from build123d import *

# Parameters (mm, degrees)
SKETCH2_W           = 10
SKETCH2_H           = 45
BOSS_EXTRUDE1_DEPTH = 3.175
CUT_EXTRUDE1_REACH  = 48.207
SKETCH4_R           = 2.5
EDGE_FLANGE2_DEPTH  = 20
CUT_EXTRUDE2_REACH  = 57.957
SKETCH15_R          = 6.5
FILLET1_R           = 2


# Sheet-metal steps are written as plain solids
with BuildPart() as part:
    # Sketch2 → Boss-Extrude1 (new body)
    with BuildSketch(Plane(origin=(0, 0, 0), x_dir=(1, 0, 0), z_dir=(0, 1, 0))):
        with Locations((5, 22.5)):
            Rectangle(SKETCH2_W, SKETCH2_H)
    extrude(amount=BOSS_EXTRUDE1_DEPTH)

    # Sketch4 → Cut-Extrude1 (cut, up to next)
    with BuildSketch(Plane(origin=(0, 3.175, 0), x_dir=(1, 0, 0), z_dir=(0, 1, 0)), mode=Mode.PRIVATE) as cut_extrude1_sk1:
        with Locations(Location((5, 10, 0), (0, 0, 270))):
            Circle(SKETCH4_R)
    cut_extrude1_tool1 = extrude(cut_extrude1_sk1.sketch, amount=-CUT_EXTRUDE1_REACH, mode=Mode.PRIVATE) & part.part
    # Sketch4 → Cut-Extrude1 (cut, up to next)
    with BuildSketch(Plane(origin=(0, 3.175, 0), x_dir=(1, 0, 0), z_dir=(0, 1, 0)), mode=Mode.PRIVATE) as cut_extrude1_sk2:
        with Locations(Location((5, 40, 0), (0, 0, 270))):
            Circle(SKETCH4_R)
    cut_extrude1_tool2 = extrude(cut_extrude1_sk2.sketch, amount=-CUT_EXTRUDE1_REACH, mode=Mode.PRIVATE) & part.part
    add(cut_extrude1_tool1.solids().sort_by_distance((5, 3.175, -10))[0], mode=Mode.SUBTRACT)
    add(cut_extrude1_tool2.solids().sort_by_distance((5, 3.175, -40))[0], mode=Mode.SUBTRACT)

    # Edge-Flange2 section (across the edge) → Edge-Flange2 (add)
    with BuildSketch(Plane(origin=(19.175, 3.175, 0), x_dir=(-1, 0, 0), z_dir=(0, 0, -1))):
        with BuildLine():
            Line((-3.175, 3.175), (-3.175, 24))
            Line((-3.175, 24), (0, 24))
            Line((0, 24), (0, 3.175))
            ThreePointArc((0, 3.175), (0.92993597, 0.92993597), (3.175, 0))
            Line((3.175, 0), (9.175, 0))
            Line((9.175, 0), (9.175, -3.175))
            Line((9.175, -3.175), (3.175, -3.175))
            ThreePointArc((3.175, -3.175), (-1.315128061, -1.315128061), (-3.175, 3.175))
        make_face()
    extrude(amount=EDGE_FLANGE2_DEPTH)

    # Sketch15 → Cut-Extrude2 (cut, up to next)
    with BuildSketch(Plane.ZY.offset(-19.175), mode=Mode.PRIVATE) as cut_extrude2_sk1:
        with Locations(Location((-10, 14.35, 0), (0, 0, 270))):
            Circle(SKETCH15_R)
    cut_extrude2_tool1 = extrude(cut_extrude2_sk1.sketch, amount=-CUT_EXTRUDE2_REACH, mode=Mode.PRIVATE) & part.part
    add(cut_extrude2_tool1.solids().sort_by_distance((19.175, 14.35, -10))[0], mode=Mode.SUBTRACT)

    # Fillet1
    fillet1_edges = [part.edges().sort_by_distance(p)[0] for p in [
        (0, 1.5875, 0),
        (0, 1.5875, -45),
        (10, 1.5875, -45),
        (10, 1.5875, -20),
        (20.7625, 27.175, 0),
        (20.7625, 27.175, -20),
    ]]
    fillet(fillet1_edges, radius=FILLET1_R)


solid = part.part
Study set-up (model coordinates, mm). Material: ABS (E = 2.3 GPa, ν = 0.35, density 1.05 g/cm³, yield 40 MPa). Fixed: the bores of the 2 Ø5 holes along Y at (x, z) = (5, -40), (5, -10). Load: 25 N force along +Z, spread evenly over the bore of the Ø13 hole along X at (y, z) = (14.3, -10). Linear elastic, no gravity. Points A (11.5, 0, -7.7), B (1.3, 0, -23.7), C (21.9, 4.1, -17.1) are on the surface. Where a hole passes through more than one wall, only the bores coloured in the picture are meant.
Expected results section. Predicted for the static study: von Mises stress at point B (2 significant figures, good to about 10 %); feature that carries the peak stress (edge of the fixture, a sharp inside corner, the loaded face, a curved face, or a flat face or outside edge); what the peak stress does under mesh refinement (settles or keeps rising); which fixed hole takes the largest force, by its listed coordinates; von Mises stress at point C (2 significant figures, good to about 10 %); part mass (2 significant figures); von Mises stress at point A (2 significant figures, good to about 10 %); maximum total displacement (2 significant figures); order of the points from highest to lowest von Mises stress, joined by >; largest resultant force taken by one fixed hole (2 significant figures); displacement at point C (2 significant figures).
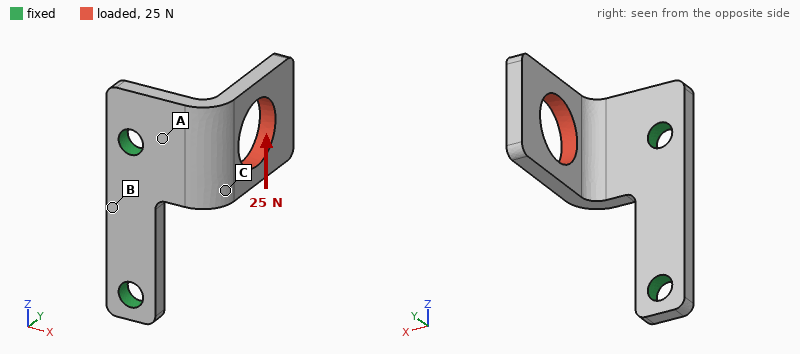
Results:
1.6 MPa
edge of the fixture
keeps rising
(5, -10)
3.3 MPa
3.2 g
5.7 MPa
0.60 mm
A > C > B
21 N
0.16 mm
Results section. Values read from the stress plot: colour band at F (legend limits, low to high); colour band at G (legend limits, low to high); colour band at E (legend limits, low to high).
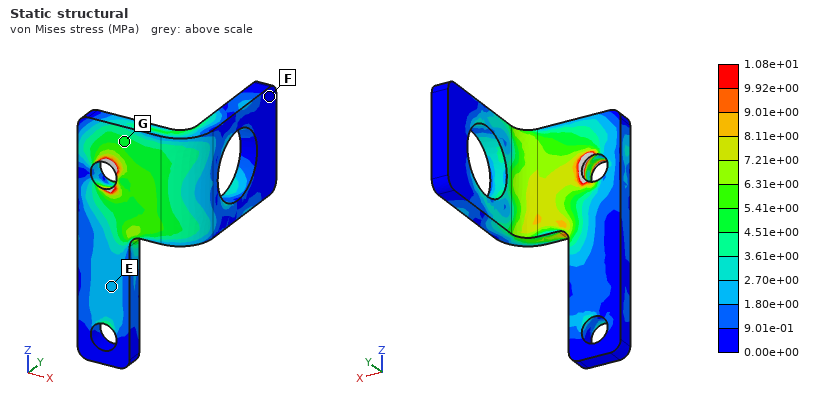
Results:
0.00e+00 to 9.01e-01 MPa
4.51e+00 to 5.41e+00 MPa
1.80e+00 to 2.70e+00 MPa
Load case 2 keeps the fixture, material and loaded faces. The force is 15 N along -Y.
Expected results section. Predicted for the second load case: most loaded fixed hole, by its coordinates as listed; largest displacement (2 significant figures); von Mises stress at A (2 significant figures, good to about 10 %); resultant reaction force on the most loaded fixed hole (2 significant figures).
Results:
(5, -10)
0.36 mm
4.0 MPa
15 N
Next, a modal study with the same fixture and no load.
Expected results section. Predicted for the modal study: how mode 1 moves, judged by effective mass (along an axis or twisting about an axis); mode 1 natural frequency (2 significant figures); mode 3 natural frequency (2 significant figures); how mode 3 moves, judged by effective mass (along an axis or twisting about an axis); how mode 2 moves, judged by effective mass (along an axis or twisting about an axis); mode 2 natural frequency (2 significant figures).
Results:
along X
660 Hz
2000 Hz
along Y
along Z
1000 Hz
